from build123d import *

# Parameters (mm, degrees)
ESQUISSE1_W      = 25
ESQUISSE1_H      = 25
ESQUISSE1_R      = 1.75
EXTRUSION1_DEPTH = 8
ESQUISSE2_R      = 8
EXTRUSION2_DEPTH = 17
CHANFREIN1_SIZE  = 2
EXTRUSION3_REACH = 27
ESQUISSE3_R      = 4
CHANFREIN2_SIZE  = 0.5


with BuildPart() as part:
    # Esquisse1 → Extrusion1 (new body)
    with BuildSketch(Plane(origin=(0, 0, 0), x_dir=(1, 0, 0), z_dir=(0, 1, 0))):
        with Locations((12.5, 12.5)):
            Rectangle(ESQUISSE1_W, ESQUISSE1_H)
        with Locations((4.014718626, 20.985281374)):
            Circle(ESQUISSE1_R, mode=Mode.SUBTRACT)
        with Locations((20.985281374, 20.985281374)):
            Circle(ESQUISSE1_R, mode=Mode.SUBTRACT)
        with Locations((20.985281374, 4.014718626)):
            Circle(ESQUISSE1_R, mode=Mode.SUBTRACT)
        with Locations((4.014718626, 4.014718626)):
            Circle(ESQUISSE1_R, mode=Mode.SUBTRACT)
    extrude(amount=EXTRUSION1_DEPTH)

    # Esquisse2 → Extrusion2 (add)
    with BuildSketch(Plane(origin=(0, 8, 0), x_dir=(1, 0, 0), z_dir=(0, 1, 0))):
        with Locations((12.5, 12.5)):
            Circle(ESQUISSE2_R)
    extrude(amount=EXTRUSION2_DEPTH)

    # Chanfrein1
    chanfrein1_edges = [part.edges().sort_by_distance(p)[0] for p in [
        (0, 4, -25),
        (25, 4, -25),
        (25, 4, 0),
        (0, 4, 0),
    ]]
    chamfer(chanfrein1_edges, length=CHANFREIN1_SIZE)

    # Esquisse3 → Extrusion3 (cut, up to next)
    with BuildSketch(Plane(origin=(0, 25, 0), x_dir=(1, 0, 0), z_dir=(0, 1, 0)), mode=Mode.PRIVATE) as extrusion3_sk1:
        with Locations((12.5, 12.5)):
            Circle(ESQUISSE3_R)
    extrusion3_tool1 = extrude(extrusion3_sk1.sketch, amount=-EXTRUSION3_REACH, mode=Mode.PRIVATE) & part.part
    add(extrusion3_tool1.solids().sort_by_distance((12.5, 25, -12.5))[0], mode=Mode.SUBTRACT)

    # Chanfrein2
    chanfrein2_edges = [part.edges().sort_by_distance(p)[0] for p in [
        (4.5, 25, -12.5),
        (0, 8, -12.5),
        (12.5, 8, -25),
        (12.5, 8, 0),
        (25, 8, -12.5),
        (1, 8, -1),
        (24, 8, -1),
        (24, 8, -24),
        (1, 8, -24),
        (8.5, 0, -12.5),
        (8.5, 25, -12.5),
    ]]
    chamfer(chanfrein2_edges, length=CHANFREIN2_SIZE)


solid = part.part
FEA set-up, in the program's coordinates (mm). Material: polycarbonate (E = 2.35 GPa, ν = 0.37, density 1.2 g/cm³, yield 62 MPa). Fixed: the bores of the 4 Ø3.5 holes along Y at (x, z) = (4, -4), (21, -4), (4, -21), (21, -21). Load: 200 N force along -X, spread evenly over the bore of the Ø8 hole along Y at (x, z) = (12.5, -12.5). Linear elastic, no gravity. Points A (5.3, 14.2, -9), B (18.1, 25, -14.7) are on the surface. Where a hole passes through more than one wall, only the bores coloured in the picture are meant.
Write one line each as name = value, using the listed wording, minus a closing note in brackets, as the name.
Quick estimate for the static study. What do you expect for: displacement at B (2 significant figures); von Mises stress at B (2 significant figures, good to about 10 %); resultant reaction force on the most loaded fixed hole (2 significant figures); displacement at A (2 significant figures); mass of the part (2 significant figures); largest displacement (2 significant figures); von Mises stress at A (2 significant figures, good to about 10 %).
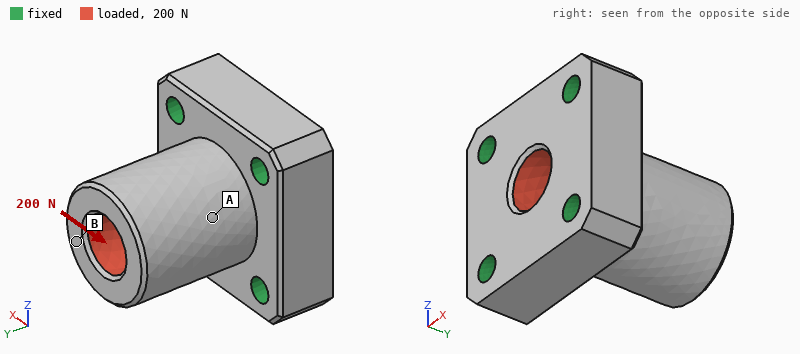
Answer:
displacement at B = 43 µm
von Mises stress at B = 0.57 MPa
resultant reaction force on the most loaded fixed hole = 73 N
displacement at A = 22 µm
mass of the part = 8.1 g
largest displacement = 44 µm
von Mises stress at A = 1.1 MPa
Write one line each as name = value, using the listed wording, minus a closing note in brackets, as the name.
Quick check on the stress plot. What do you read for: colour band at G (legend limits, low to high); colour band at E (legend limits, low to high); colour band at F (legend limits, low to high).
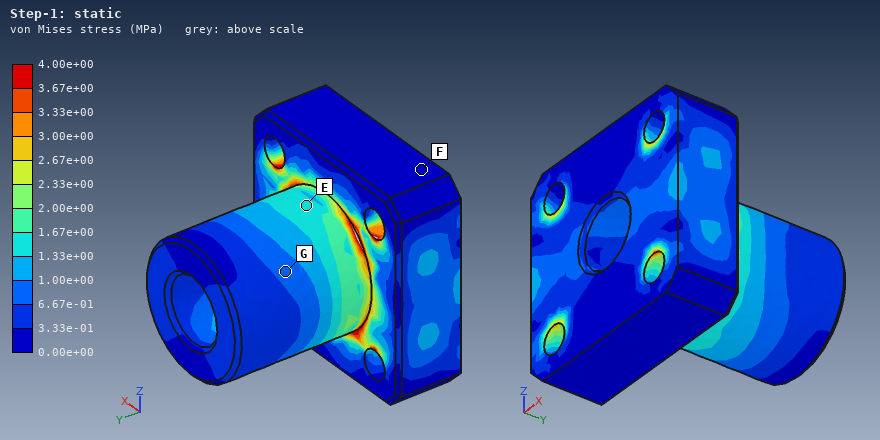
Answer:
colour band at G = 6.67e-01 to 1.00e+00 MPa
colour band at E = 1.33e+00 to 1.67e+00 MPa
colour band at F = 0.00e+00 to 3.33e-01 MPa
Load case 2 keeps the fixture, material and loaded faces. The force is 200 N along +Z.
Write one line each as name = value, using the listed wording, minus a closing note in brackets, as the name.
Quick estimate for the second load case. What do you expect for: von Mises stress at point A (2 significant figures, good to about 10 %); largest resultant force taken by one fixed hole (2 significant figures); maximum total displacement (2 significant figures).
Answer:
von Mises stress at point A = 1.3 MPa
largest resultant force taken by one fixed hole = 73 N
maximum total displacement = 44 µm
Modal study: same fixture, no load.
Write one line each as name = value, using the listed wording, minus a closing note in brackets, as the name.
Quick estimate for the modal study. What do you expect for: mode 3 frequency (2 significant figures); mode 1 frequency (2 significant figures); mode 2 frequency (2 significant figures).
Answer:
mode 3 frequency = 11 kHz
mode 1 frequency = 5900 Hz
mode 2 frequency = 5900 Hz
